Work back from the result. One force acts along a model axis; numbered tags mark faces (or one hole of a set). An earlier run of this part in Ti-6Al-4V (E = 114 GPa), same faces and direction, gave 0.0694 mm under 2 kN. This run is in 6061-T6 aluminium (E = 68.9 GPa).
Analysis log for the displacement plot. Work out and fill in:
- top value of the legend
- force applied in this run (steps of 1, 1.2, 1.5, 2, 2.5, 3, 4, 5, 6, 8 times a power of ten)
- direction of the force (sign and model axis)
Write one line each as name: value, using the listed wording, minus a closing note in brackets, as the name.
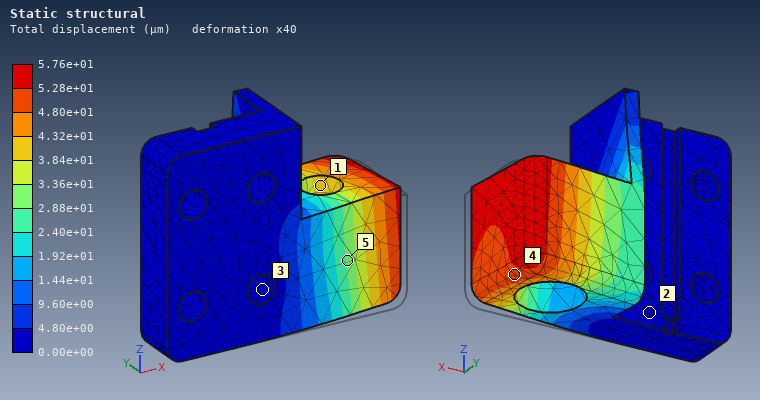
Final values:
top value of the legend: 5.76e+01 µm
force applied in this run: 1 kN
direction of the force: +Y
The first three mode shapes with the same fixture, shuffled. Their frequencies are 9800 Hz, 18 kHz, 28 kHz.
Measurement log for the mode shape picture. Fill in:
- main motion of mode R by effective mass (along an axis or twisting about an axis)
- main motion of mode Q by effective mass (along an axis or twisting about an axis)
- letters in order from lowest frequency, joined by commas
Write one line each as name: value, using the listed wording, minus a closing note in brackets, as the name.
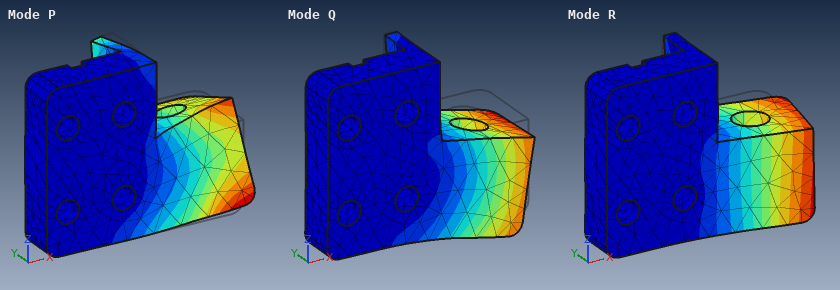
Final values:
main motion of mode R by effective mass: along Y
main motion of mode Q by effective mass: along Z
letters in order from lowest frequency, joined by commas: R, Q, P
